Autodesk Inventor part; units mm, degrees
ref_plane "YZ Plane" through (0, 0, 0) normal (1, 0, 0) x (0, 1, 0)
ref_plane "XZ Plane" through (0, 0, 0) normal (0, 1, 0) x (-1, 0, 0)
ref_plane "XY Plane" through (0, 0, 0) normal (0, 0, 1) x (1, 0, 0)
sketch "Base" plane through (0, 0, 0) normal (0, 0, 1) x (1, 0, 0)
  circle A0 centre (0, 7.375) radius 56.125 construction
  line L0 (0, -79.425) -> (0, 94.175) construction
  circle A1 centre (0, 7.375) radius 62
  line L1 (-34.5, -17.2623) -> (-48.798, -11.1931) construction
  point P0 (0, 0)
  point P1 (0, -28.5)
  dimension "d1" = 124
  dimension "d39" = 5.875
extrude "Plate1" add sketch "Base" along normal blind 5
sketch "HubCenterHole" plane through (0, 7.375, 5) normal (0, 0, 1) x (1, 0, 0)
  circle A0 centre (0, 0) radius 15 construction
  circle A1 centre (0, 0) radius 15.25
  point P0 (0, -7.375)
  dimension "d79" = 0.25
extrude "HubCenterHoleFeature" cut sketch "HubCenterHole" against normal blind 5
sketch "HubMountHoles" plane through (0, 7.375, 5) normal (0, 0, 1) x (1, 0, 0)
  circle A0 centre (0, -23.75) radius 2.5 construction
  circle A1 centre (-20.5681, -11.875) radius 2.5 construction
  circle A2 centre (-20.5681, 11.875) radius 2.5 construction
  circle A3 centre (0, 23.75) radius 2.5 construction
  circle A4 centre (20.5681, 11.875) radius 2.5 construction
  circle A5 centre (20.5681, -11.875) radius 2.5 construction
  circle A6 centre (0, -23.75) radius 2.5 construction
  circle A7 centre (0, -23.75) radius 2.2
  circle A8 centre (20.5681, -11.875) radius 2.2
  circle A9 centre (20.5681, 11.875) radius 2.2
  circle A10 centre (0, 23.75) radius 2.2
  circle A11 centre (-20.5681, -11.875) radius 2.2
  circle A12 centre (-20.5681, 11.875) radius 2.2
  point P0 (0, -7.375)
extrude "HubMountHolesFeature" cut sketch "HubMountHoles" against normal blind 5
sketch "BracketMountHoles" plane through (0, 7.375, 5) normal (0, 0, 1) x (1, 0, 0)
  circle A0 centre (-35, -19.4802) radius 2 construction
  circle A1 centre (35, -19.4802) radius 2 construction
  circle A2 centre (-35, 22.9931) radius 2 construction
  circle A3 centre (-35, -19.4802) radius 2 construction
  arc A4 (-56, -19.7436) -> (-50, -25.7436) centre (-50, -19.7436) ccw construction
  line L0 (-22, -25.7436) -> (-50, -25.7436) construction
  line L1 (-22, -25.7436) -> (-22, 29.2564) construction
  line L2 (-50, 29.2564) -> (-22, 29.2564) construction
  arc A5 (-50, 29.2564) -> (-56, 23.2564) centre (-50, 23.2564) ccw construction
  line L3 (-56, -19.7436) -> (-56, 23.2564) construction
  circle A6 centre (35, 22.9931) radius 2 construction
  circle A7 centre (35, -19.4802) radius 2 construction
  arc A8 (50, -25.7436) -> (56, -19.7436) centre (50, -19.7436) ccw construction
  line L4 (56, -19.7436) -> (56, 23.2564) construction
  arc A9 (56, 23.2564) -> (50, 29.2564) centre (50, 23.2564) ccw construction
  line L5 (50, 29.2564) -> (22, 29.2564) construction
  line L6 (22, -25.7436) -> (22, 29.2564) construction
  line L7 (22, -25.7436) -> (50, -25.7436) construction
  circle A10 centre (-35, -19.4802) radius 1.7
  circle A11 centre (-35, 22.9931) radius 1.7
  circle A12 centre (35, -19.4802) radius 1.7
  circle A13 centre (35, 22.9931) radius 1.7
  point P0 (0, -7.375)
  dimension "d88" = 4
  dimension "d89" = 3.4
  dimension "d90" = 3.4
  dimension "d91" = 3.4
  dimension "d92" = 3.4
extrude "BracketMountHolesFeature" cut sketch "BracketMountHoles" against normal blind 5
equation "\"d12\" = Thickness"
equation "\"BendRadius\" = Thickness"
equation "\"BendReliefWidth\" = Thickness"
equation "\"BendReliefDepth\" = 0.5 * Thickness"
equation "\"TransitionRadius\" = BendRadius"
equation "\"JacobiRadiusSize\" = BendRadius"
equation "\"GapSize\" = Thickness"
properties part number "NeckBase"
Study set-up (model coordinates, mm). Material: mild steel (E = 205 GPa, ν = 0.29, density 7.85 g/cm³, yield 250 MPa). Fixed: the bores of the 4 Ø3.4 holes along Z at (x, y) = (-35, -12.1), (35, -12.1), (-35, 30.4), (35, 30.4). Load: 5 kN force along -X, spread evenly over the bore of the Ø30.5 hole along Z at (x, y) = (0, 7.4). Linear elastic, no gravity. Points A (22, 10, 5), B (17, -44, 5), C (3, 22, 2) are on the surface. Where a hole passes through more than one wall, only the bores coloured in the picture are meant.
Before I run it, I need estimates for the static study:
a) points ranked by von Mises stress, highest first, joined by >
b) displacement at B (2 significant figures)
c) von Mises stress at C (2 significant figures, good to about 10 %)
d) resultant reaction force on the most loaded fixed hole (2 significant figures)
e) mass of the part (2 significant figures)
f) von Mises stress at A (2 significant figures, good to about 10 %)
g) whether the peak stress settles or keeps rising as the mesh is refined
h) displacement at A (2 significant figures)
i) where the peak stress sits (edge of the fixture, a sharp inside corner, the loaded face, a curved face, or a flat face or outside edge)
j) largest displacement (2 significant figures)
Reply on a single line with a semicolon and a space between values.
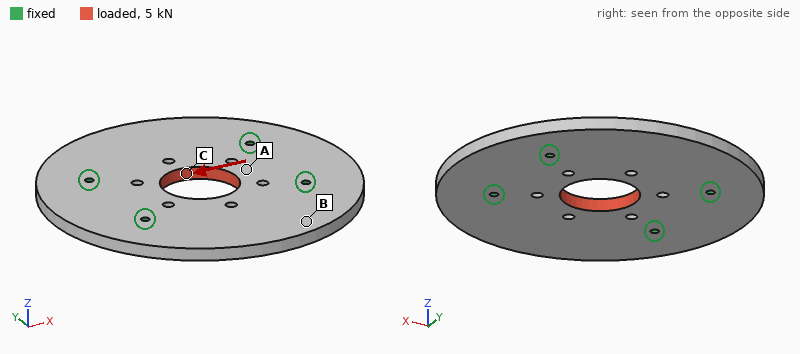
C > A > B; 0.70 µm; 18 MPa; 1.3 kN; 440 g; 8.2 MPa; keeps rising; 1.5 µm; edge of the fixture; 1.9 µm
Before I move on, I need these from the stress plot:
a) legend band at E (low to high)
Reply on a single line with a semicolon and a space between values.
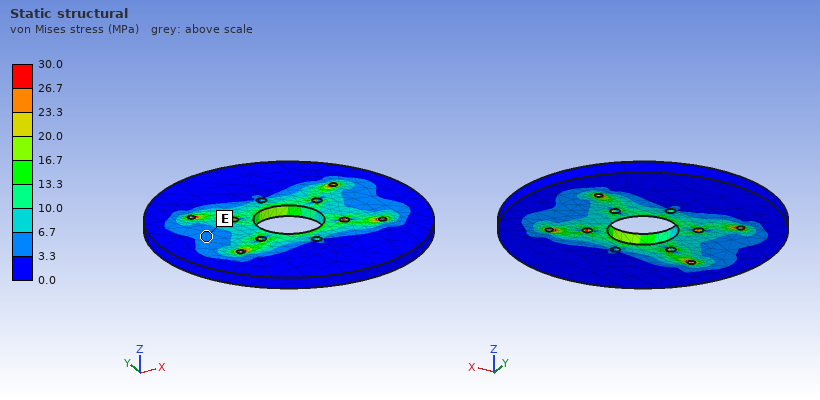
3.3 to 6.7 MPa
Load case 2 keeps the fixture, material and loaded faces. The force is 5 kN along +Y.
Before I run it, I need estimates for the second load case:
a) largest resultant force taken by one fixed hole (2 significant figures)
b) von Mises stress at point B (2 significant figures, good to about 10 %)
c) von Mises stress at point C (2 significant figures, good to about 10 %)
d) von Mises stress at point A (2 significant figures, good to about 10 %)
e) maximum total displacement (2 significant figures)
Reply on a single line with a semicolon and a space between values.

1.3 kN; 4.6 MPa; 9.6 MPa; 15 MPa; 3.0 µm
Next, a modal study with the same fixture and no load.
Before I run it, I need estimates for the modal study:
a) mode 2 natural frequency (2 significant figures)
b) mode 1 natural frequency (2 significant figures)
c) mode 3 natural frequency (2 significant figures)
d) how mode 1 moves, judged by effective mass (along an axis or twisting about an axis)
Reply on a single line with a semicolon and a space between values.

2400 Hz; 2100 Hz; 4700 Hz; along Z
